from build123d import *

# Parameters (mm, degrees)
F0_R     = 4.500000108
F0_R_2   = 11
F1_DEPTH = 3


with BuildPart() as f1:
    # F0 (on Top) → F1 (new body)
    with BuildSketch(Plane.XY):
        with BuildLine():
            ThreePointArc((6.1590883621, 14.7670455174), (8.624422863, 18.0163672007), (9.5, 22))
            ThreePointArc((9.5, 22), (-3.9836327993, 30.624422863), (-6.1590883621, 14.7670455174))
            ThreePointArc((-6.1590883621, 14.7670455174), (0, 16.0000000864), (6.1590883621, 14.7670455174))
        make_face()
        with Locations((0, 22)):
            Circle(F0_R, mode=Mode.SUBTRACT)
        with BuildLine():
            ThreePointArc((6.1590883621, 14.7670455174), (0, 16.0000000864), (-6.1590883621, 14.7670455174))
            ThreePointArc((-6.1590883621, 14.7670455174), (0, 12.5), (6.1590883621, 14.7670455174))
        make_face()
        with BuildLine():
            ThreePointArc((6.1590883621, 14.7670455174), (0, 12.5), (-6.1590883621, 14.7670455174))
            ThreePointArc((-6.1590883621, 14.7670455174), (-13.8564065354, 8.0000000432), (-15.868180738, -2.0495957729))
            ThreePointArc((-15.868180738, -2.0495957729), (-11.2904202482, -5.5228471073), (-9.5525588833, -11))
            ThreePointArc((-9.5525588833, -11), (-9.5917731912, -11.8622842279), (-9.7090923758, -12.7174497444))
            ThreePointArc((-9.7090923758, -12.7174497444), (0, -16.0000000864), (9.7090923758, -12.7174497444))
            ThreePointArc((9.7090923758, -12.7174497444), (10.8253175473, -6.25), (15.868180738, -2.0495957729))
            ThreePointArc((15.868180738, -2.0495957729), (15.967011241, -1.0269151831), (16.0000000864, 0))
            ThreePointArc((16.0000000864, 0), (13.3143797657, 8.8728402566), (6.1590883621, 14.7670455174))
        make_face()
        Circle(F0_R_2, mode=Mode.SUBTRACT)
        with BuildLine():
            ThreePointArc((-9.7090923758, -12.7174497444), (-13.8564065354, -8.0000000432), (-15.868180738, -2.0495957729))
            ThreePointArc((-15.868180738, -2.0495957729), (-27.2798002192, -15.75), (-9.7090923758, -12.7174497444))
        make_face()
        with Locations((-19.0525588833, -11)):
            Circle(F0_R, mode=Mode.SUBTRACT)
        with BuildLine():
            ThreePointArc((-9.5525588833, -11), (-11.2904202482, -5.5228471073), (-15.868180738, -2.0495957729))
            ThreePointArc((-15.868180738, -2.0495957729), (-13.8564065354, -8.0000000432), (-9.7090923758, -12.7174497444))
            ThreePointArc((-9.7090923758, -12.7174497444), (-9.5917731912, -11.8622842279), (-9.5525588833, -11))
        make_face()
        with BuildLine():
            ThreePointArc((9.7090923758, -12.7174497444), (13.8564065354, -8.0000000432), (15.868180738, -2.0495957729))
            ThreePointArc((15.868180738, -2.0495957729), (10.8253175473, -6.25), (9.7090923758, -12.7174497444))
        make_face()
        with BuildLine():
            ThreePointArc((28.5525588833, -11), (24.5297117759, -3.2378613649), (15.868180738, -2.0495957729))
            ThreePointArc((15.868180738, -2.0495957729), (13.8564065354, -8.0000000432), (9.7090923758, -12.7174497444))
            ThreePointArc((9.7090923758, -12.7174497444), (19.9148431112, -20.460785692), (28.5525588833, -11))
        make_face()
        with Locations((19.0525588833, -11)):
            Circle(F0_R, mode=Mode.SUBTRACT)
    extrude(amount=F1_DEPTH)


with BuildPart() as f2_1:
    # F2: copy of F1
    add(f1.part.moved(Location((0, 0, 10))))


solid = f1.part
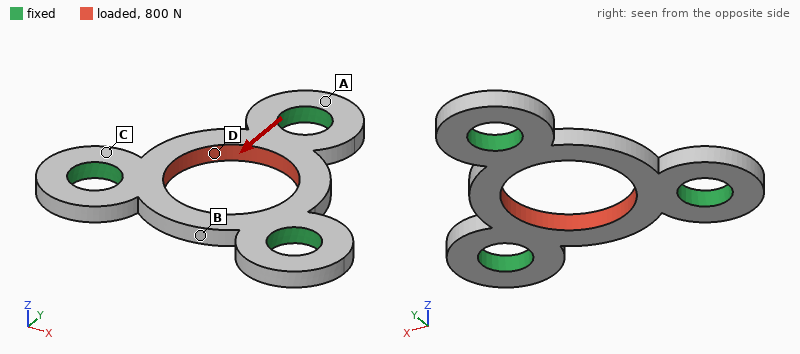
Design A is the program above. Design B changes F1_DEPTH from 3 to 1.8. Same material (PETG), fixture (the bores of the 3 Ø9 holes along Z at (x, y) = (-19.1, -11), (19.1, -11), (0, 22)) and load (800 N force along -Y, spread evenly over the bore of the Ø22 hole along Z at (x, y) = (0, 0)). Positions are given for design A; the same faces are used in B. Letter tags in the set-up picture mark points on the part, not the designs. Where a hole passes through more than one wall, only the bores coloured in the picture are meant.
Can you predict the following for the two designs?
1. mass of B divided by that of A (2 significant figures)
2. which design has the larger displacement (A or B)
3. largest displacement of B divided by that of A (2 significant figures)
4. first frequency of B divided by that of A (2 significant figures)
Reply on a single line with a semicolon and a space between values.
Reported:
0.60; B; 1.7; 0.65
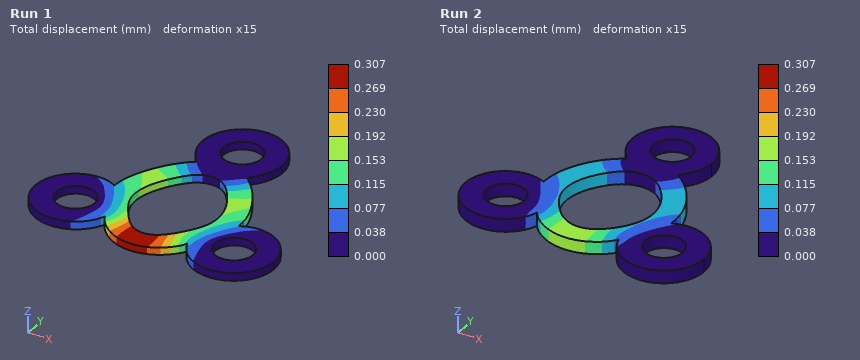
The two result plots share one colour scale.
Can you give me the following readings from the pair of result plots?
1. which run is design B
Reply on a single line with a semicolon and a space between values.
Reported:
Run 1
